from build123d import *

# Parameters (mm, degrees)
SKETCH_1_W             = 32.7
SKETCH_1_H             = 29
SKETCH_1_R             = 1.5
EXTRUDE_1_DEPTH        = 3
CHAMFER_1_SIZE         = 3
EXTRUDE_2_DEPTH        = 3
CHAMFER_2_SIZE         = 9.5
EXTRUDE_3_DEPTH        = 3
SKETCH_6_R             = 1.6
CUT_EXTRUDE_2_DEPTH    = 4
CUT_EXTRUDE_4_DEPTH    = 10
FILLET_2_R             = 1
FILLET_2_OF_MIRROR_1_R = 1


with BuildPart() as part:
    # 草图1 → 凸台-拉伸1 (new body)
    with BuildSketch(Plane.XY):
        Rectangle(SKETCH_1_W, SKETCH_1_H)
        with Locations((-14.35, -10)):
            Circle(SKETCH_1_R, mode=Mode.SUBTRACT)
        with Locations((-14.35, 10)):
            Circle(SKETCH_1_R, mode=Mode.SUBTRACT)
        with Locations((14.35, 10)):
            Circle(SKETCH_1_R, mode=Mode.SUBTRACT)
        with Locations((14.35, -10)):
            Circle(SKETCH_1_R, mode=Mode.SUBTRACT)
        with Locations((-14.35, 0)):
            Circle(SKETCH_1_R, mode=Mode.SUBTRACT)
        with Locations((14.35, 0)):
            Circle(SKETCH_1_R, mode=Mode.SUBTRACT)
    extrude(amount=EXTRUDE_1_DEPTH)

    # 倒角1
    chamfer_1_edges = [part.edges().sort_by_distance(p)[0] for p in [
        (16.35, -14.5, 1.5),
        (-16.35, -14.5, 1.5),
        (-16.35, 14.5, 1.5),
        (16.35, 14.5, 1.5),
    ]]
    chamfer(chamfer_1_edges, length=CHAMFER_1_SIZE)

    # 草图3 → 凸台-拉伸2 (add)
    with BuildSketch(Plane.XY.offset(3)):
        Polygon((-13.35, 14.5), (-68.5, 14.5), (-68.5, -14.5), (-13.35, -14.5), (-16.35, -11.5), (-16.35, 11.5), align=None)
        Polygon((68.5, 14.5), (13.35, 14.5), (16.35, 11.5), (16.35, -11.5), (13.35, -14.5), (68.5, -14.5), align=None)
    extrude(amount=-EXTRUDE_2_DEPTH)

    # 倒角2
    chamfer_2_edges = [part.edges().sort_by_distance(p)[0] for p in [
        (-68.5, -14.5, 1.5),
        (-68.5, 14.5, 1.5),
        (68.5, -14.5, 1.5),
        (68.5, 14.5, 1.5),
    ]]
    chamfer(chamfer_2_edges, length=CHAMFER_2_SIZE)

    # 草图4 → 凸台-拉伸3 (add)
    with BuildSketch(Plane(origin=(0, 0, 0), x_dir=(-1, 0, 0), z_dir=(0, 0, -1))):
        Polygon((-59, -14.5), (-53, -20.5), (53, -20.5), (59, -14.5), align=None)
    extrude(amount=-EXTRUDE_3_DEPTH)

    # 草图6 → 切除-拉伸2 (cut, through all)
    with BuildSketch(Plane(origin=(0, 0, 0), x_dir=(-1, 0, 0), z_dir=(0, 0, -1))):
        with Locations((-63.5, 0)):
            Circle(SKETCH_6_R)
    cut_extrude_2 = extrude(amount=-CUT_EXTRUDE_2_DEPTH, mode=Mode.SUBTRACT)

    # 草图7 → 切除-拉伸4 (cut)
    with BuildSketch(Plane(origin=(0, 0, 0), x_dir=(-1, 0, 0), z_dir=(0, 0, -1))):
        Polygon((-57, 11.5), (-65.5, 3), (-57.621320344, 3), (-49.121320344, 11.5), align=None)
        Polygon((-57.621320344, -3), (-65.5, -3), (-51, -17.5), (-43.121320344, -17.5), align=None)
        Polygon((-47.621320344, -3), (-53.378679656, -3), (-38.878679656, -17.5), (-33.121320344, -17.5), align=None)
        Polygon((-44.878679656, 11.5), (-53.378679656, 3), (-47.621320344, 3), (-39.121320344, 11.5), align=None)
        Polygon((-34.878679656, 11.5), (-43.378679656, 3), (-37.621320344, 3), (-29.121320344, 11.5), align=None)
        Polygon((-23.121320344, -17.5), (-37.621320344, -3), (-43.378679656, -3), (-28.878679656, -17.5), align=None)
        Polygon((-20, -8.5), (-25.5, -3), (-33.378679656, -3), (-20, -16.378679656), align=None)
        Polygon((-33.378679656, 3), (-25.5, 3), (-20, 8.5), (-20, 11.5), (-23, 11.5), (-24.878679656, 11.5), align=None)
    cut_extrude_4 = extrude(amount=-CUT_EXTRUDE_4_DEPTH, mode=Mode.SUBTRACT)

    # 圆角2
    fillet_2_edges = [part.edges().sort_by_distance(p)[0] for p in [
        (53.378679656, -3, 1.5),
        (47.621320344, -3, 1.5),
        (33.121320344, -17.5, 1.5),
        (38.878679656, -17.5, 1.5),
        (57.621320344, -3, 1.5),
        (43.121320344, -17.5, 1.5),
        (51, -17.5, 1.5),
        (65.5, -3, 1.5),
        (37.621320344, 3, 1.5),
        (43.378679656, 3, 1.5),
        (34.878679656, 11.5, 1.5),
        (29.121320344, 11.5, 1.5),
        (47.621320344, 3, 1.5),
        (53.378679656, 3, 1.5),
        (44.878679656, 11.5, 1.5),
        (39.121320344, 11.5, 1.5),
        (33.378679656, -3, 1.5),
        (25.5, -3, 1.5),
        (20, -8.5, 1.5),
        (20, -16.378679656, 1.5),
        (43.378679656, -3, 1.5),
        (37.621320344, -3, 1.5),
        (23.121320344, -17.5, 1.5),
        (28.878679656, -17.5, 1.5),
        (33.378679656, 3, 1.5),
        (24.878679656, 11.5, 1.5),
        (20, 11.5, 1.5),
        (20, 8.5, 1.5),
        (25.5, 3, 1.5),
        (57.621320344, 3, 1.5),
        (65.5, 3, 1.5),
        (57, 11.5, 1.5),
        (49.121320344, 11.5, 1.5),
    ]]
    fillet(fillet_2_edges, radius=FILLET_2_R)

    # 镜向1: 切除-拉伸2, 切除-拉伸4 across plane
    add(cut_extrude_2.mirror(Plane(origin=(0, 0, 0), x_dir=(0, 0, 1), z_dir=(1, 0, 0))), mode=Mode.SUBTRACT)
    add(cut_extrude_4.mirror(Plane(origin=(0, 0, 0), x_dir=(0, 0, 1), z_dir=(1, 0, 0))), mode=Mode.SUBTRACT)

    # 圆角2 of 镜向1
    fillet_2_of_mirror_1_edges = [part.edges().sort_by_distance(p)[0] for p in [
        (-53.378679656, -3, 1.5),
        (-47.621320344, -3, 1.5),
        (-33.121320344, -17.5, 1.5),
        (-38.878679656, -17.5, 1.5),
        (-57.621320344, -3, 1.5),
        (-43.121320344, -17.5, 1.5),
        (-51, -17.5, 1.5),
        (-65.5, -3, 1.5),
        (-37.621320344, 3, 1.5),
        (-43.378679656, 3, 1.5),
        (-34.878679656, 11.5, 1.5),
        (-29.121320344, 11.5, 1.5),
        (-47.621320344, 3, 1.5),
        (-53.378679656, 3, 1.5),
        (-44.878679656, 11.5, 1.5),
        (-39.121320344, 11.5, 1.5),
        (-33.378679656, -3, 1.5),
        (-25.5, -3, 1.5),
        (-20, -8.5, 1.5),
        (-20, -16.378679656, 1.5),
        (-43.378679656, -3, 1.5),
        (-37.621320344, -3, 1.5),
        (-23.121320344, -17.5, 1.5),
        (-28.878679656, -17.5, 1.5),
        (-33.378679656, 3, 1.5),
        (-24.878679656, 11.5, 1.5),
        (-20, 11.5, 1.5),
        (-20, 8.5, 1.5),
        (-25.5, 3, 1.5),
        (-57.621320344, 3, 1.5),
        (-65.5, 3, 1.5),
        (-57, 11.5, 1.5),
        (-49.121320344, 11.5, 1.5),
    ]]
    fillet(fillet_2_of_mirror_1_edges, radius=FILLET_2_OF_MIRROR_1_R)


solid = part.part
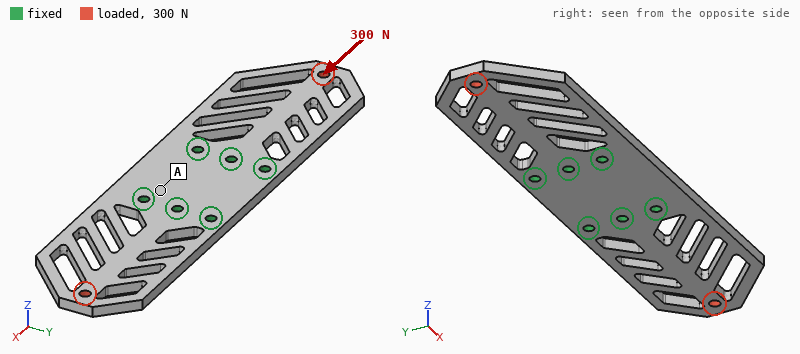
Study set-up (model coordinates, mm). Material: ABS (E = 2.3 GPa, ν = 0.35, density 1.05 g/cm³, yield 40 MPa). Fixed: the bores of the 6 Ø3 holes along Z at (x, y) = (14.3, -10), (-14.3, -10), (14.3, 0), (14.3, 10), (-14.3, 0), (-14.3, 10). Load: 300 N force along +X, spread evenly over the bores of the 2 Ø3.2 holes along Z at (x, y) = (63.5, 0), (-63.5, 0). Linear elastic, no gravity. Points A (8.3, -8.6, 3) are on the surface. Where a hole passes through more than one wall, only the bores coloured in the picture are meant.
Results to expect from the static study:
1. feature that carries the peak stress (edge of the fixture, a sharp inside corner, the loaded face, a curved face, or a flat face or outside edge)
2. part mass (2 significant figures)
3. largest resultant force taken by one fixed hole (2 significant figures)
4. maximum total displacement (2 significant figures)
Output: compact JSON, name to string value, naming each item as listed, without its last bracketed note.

{"feature that carries the peak stress": "the loaded face", "part mass": "10 g", "largest resultant force taken by one fixed hole": "58 N", "maximum total displacement": "0.13 mm"}
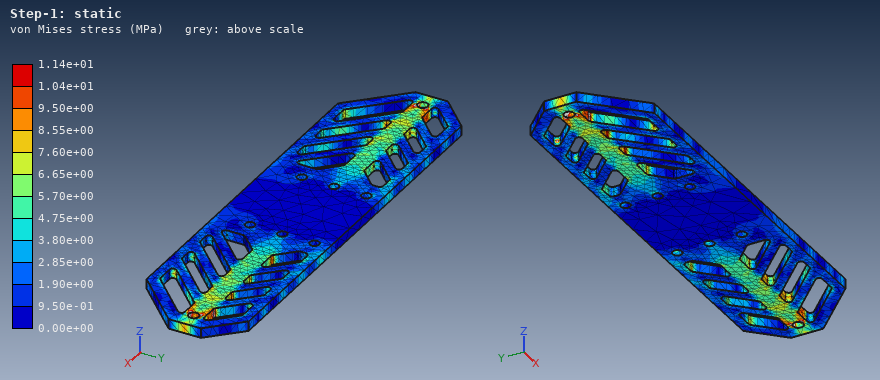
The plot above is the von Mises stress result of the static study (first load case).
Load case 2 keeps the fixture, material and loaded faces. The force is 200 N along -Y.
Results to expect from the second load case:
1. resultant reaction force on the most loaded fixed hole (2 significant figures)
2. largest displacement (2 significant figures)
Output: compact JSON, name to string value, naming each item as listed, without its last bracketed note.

{"resultant reaction force on the most loaded fixed hole": "170 N", "largest displacement": "0.94 mm"}
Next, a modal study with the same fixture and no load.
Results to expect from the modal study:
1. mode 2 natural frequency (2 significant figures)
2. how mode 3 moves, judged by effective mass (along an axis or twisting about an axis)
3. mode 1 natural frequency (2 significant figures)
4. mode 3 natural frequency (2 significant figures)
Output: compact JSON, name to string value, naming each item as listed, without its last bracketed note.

{"mode 2 natural frequency": "270 Hz", "how mode 3 moves, judged by effective mass": "twisting about X", "mode 1 natural frequency": "260 Hz", "mode 3 natural frequency": "830 Hz"}
